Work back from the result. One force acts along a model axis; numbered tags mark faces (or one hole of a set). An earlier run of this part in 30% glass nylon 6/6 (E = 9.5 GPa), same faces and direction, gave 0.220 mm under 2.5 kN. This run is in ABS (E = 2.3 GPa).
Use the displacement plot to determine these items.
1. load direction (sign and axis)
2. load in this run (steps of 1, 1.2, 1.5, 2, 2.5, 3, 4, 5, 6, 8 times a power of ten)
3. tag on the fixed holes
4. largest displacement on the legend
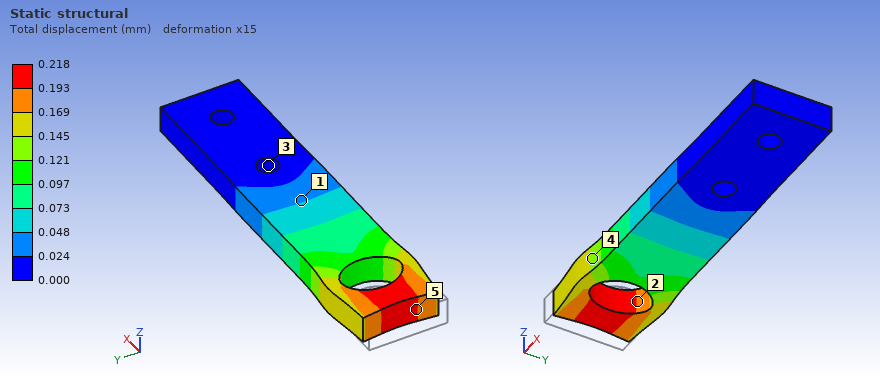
+X
600 N
3
0.218 mm
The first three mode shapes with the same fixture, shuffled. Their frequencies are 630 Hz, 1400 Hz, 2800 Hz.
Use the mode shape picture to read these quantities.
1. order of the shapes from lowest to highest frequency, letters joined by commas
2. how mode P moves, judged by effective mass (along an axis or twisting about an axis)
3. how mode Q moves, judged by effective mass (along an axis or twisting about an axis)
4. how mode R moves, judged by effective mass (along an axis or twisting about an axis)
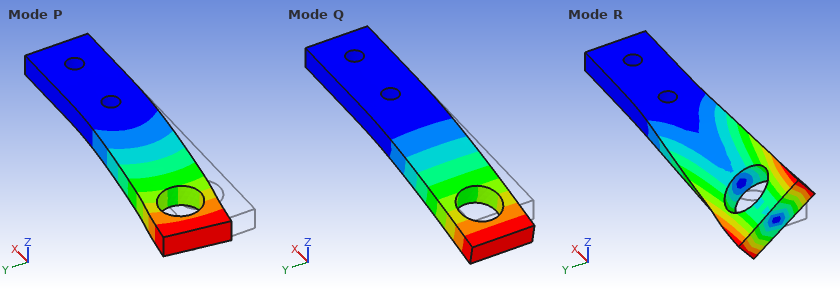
Q, P, R
along Y
along Z
twisting about X
